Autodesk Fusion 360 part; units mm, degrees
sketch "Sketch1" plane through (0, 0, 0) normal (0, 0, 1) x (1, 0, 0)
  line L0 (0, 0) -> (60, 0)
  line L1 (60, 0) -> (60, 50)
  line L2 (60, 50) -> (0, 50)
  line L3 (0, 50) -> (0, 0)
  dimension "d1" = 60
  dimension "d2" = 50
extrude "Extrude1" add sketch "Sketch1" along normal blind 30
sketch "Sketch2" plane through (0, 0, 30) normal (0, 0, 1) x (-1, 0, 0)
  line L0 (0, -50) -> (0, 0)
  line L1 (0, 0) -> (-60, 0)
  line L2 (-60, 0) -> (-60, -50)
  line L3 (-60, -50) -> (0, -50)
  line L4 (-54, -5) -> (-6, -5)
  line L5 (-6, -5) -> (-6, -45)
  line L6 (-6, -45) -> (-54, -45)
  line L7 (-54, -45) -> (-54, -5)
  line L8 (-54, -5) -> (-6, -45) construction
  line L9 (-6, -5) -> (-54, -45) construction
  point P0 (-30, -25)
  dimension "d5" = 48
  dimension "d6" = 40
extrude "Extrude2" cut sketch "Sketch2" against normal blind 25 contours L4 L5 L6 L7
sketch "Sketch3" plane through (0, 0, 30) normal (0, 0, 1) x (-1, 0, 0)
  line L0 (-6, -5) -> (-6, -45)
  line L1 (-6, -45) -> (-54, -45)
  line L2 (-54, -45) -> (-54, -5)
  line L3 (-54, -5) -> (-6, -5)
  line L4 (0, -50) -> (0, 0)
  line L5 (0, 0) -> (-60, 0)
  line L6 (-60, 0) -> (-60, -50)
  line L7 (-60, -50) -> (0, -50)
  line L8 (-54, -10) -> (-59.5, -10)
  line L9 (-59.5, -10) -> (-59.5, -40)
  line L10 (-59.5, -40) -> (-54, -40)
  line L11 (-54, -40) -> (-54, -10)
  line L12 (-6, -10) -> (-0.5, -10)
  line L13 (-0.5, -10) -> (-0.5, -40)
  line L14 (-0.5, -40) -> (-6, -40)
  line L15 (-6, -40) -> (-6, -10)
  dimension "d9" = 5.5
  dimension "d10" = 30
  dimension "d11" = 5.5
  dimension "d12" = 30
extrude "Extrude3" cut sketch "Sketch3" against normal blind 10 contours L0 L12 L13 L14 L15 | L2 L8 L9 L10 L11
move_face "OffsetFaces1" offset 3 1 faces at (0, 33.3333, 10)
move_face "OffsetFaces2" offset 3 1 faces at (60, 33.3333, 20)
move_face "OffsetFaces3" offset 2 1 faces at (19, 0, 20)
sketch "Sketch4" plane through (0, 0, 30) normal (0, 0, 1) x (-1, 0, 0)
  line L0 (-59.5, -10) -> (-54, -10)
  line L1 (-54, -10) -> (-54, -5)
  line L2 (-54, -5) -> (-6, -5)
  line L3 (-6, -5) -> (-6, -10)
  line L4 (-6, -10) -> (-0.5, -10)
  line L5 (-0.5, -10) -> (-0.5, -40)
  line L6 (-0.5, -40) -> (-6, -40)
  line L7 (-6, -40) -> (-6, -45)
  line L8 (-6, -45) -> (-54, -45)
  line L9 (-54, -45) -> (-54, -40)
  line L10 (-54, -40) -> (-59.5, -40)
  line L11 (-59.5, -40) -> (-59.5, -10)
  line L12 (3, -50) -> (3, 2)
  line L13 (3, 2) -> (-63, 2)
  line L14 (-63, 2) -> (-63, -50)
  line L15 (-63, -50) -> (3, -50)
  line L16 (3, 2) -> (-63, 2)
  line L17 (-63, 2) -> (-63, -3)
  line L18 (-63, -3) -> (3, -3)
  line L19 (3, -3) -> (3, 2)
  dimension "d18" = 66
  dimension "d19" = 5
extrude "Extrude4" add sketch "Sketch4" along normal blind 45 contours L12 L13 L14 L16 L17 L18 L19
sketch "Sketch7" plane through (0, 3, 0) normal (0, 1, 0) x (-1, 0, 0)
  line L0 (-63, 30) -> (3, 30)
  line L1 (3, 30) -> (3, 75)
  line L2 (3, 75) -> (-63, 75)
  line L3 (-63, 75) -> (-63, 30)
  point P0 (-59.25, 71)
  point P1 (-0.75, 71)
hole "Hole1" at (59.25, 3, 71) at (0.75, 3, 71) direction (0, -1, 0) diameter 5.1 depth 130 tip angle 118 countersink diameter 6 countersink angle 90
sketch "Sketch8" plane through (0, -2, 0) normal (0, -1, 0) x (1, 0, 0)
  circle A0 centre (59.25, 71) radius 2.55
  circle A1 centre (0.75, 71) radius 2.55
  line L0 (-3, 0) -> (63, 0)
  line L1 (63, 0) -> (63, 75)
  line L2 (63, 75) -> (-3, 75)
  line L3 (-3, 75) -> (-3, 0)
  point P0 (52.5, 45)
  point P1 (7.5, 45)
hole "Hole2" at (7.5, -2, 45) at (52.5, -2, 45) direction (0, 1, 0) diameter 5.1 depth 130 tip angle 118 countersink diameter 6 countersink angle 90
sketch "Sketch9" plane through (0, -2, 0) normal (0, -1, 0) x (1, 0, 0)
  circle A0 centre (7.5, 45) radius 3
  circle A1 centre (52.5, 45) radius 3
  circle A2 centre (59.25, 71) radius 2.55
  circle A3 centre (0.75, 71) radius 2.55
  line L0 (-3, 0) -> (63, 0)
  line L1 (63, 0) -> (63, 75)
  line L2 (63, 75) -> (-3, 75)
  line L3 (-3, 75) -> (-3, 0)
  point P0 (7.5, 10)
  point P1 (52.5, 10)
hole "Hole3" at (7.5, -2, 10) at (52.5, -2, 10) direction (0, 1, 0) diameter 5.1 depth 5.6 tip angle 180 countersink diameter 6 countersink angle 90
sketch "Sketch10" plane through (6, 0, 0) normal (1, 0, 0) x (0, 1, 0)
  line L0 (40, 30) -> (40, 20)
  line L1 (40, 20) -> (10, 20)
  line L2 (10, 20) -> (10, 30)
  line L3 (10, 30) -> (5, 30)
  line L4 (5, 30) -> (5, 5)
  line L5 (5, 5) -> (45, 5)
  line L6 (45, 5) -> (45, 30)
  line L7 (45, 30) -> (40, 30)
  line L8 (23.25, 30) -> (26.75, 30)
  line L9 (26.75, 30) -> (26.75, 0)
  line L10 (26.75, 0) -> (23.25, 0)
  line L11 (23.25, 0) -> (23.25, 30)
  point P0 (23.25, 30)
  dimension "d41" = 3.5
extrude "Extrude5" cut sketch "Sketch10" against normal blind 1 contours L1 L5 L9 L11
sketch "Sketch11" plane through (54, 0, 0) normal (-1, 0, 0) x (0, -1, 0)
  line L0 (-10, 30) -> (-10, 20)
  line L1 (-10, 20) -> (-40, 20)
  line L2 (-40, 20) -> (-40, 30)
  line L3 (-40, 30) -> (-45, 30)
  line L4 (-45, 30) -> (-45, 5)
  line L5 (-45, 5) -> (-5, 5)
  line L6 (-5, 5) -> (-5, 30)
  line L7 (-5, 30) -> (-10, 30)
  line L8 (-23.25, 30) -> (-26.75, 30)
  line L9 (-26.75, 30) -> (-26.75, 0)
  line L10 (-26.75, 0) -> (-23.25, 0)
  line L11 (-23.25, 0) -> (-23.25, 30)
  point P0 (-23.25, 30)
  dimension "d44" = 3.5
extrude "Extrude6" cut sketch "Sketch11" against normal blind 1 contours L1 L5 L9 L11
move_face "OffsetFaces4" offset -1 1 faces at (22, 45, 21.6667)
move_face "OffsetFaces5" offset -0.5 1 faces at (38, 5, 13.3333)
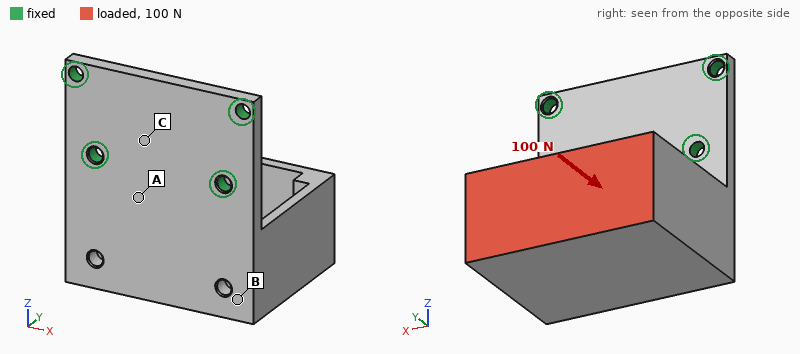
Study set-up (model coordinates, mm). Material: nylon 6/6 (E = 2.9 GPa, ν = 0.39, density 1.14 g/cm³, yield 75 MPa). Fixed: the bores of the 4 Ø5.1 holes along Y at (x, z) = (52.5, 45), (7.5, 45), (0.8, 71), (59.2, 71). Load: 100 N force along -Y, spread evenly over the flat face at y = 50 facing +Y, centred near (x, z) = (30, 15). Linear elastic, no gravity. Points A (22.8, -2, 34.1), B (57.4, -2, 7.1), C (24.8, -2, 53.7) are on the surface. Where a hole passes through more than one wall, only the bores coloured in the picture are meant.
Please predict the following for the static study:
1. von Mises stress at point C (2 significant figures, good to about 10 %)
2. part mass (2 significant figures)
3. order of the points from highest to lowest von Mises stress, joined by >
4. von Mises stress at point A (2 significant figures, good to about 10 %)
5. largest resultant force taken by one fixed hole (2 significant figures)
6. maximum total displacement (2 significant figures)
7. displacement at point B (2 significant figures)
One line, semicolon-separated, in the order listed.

2.2 MPa; 73 g; A > C > B; 5.4 MPa; 67 N; 1.2 mm; 0.61 mm
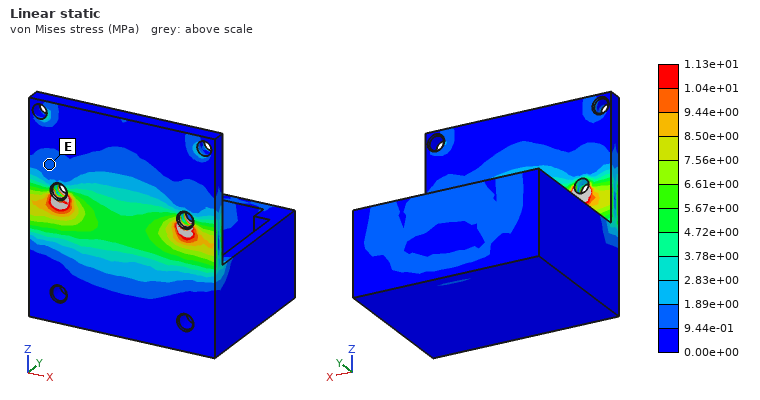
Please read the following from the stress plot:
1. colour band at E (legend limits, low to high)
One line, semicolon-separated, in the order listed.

9.44e-01 to 1.89e+00 MPa
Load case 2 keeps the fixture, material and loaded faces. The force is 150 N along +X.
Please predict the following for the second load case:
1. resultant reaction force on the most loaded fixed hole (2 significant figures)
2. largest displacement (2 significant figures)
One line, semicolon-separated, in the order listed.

190 N; 1.3 mm
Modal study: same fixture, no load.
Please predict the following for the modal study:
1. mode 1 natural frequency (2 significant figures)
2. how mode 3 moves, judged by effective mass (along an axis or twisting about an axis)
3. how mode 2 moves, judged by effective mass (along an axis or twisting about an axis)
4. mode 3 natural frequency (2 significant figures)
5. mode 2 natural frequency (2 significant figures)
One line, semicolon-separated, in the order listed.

180 Hz; along Y; along X; 1000 Hz; 390 Hz
